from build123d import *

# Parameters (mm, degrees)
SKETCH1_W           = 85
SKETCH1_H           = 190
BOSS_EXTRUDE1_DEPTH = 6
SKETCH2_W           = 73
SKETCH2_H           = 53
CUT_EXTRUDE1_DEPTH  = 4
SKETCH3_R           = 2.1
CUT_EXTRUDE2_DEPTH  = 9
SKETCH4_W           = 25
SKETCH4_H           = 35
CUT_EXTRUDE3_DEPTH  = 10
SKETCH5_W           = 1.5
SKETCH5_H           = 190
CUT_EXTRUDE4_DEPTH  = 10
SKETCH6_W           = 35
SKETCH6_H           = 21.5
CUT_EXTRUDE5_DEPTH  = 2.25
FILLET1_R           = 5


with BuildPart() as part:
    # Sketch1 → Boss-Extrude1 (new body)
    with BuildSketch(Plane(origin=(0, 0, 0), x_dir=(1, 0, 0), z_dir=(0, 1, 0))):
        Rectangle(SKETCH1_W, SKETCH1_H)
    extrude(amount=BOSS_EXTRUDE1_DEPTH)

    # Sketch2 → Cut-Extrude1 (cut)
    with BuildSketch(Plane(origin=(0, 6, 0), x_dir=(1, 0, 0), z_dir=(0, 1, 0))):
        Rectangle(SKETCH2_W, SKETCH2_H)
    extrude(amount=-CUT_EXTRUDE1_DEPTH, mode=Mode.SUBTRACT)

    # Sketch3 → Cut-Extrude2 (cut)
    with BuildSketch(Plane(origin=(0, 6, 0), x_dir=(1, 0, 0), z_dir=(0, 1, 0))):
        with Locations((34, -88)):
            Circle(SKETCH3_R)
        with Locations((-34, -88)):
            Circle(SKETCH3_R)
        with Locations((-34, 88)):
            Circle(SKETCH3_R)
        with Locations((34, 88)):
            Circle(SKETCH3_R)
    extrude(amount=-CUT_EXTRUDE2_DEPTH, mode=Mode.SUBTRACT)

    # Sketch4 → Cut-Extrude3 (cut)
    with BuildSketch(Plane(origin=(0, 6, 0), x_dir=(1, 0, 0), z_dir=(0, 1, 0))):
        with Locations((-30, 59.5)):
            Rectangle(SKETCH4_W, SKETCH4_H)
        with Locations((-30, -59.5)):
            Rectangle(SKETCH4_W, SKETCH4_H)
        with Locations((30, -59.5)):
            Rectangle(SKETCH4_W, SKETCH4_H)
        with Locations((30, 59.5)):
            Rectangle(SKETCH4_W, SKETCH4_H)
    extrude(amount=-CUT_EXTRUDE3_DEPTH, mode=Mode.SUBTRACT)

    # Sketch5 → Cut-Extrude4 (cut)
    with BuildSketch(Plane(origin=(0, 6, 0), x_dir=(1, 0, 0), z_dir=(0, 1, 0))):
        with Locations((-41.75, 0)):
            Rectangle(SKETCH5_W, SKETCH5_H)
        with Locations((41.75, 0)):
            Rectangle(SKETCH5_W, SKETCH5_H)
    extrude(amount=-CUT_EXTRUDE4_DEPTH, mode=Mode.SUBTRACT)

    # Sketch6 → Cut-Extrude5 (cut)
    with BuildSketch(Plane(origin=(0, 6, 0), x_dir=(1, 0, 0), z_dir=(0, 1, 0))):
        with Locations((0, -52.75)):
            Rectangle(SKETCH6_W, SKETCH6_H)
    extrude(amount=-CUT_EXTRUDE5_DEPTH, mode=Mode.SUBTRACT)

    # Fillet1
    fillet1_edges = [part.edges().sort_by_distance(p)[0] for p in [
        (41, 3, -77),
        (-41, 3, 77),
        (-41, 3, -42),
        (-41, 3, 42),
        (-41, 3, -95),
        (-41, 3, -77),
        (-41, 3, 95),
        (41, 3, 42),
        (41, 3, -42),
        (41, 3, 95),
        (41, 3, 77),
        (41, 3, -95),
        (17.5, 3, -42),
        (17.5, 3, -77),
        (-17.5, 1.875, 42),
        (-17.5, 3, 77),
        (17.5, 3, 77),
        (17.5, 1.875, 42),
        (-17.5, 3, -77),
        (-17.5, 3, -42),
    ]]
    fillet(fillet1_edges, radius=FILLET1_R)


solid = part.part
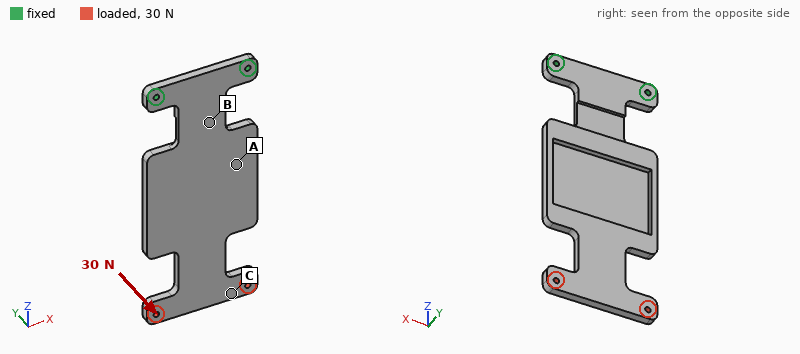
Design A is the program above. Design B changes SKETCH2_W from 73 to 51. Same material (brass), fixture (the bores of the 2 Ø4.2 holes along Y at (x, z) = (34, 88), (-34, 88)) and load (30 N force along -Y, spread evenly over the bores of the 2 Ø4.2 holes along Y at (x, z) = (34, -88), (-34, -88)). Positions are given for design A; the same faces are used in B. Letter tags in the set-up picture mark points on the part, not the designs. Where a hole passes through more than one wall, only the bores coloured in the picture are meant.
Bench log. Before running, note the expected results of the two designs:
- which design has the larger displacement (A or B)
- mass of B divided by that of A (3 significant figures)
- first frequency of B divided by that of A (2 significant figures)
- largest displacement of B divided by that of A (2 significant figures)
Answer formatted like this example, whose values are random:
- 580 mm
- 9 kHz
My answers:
- A
- 1.08
- 1.0
- 0.86
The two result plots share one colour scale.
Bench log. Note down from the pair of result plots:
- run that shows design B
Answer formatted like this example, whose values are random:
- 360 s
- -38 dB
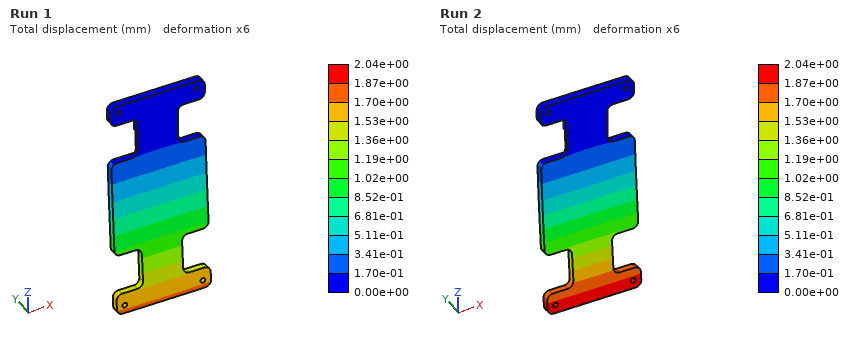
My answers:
- Run 1
